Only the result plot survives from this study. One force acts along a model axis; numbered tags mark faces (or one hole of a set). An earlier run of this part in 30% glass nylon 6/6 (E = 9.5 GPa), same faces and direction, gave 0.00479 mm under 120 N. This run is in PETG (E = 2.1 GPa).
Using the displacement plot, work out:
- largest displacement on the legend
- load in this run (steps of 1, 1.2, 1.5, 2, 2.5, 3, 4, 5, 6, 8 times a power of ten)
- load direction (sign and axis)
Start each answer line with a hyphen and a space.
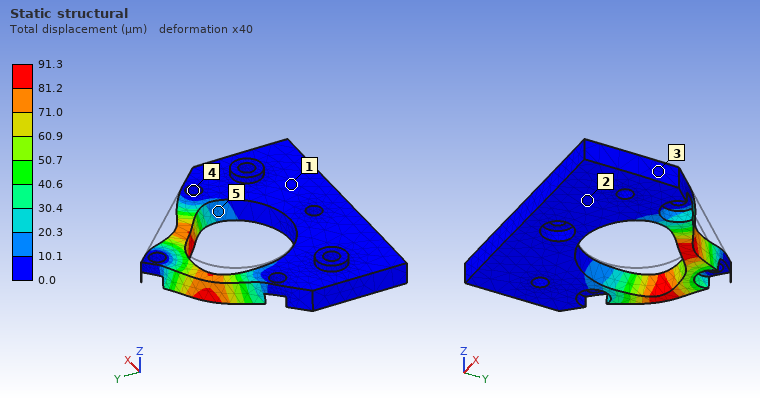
- 91.3 µm
- 500 N
- -X
